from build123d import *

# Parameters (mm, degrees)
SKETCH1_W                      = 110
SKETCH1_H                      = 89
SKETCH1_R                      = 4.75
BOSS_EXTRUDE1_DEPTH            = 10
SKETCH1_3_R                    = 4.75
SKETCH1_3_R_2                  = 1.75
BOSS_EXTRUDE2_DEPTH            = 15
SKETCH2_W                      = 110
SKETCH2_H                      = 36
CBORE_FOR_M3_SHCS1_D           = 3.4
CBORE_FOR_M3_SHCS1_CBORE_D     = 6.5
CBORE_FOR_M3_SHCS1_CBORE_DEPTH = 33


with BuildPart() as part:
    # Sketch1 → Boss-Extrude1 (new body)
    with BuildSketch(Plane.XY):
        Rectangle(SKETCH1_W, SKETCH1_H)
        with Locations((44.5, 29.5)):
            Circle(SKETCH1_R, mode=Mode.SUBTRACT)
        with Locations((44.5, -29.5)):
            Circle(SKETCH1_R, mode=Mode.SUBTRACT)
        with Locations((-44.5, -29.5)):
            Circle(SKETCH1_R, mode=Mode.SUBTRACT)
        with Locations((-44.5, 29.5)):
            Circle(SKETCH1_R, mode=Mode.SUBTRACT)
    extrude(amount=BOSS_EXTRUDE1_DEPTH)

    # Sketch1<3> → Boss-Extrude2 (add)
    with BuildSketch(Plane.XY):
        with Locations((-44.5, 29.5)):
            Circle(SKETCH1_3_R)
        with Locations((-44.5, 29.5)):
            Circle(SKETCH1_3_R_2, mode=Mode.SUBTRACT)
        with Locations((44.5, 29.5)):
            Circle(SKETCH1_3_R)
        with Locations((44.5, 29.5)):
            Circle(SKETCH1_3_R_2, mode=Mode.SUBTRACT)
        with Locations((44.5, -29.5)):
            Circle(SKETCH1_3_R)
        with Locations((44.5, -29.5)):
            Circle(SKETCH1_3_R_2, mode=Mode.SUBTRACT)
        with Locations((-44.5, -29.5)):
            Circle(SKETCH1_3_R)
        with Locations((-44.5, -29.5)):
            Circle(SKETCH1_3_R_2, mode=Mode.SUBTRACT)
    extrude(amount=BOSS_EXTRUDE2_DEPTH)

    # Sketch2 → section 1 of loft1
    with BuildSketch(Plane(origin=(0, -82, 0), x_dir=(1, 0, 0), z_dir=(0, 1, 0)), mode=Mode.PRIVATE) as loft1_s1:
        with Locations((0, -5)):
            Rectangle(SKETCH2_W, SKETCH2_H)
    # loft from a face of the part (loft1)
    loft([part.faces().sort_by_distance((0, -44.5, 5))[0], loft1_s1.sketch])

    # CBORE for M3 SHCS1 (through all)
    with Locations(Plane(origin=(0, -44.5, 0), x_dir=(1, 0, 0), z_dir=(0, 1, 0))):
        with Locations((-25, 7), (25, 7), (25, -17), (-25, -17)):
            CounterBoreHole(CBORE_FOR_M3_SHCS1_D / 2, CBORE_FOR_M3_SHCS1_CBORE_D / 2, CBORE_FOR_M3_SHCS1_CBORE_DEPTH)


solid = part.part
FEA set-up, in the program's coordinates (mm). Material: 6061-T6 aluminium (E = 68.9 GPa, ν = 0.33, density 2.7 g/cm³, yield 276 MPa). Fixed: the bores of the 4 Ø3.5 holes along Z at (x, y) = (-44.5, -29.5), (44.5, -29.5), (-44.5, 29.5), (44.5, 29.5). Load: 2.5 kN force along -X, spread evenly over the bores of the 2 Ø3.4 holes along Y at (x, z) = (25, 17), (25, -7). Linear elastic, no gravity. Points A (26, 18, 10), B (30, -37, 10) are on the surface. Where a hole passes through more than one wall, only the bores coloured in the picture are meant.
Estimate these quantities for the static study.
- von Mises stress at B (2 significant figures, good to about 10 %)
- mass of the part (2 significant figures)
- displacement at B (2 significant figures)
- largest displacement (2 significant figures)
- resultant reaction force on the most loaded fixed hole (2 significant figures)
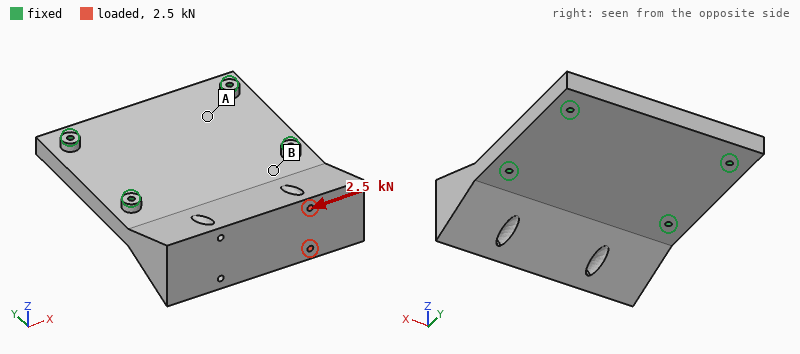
5.1 MPa
520 g
1.7 µm
9.5 µm
1.7 kN
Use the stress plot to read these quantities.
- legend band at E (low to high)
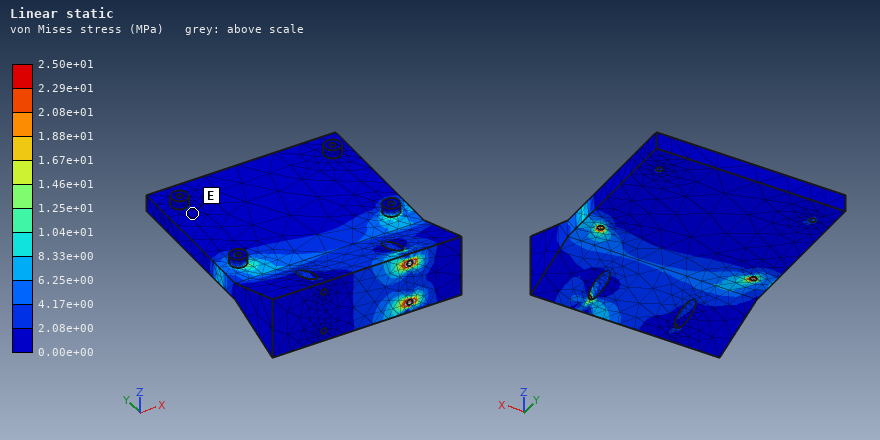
0.00e+00 to 2.08e+00 MPa
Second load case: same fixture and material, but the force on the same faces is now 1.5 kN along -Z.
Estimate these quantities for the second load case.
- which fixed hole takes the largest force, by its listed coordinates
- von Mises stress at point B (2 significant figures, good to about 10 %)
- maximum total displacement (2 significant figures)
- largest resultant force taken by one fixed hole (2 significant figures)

(44.5, -29.5)
30 MPa
0.15 mm
1.5 kN
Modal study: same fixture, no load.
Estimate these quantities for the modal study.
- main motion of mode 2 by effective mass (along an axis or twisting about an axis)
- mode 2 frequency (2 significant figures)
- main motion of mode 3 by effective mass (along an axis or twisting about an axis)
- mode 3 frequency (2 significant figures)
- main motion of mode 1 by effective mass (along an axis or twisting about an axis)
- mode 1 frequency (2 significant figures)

twisting about Y
4000 Hz
along Z
5200 Hz
along Z
1500 Hz
